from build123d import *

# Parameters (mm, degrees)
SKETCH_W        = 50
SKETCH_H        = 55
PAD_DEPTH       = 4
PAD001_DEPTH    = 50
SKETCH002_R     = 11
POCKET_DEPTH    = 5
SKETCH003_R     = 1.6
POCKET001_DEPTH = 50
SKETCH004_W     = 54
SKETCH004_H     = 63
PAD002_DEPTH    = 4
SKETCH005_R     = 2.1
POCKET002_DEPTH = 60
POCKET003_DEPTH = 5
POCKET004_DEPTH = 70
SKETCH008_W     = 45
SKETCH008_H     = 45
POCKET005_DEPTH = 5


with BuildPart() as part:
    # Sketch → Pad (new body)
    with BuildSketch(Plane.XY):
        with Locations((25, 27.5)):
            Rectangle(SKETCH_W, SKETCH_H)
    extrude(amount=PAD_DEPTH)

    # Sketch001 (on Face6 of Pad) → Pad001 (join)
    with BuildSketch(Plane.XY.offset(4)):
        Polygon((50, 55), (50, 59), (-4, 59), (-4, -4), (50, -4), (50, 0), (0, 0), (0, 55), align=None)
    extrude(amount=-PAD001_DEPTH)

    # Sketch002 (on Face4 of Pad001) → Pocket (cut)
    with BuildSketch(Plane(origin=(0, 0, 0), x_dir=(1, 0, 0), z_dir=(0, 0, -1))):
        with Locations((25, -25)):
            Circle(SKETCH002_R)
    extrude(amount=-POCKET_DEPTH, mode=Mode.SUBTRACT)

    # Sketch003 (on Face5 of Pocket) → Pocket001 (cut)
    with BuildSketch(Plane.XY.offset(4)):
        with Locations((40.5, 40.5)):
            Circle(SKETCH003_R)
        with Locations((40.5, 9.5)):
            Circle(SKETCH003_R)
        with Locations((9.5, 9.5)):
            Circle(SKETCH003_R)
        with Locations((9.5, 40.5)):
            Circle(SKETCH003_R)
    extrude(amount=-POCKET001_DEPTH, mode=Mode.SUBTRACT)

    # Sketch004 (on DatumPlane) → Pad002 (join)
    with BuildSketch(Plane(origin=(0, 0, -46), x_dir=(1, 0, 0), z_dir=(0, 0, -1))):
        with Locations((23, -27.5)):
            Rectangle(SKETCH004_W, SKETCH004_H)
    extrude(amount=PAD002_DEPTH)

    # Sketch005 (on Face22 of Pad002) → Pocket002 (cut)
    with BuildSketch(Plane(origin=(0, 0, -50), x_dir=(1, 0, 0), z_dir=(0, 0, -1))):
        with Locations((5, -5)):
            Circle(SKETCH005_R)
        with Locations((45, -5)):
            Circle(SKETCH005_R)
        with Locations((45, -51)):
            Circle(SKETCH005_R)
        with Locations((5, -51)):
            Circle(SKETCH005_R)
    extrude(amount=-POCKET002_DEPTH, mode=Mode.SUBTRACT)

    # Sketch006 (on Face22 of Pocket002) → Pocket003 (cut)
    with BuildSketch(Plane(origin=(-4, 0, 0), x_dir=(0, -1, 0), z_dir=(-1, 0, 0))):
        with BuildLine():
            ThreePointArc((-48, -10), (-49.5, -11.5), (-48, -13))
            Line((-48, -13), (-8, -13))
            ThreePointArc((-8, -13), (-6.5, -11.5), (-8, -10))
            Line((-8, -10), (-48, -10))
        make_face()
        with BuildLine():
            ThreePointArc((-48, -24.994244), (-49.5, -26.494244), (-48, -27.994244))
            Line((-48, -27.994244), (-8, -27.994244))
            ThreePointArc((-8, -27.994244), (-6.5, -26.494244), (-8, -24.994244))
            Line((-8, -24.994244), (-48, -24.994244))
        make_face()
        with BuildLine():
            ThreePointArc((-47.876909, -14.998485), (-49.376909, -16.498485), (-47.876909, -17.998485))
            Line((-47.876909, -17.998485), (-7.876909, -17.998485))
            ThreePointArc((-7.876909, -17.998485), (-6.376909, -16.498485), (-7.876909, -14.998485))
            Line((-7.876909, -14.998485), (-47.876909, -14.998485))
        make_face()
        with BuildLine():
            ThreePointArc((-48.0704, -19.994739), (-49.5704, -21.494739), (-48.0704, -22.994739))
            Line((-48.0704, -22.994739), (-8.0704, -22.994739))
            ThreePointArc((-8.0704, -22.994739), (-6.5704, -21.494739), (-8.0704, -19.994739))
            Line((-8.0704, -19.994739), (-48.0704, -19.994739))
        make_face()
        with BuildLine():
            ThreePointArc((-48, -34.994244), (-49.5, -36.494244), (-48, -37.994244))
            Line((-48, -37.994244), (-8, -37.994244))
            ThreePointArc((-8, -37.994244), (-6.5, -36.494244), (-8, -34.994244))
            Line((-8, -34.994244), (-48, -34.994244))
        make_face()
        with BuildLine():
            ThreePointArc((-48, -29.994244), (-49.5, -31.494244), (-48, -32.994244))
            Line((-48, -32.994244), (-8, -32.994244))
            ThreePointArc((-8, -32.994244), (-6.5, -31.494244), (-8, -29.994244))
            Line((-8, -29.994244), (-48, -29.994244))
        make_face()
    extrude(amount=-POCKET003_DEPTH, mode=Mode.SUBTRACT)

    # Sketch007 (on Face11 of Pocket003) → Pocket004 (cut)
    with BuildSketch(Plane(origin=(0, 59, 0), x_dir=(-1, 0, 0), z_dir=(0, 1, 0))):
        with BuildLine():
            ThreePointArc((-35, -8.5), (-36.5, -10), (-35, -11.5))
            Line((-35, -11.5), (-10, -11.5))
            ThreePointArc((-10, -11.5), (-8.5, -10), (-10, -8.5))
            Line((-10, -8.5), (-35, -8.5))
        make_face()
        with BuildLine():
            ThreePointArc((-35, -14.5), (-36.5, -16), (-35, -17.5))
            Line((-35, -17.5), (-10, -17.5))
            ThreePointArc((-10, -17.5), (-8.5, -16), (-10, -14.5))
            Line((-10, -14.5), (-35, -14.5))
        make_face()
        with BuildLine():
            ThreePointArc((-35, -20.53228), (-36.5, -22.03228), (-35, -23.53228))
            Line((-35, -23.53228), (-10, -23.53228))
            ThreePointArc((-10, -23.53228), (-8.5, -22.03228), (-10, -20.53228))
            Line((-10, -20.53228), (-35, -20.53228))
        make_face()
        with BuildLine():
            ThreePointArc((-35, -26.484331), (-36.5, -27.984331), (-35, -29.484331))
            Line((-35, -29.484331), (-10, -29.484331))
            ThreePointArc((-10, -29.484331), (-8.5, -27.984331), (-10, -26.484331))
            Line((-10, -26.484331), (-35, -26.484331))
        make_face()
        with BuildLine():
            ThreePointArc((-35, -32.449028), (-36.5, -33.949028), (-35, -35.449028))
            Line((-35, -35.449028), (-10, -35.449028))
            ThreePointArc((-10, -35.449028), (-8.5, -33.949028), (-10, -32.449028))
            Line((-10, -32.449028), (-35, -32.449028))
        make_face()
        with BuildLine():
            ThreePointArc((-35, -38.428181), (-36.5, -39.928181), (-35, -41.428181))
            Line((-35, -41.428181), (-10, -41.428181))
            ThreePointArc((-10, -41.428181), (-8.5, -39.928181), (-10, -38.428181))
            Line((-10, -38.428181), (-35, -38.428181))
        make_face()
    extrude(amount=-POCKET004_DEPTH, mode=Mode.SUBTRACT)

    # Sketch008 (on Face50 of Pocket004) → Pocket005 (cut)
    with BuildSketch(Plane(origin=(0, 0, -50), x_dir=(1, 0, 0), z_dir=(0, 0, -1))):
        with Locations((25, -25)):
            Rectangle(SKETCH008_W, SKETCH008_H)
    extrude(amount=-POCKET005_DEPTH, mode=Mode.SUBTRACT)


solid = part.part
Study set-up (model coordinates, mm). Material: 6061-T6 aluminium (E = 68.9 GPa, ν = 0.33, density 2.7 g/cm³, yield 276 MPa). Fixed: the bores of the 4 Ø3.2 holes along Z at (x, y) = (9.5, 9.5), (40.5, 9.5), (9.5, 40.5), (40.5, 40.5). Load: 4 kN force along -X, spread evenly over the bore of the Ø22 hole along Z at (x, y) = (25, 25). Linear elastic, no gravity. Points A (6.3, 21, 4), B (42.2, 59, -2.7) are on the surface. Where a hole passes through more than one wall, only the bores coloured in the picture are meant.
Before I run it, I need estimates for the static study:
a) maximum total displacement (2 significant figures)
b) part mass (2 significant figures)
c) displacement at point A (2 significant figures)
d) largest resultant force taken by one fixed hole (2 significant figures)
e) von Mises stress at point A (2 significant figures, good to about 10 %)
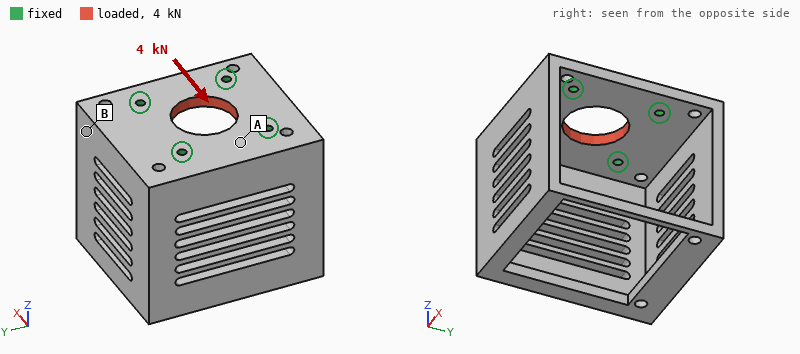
7.0 µm
110 g
4.0 µm
1.0 kN
10 MPa
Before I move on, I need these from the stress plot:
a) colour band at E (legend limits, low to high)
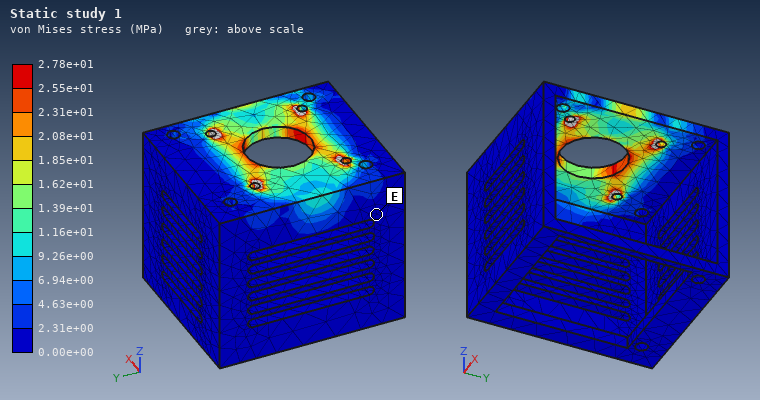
0.00e+00 to 2.31e+00 MPa
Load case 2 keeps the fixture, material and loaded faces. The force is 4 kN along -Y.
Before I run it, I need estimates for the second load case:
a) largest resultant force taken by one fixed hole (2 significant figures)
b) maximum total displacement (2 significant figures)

1.0 kN
5.8 µm
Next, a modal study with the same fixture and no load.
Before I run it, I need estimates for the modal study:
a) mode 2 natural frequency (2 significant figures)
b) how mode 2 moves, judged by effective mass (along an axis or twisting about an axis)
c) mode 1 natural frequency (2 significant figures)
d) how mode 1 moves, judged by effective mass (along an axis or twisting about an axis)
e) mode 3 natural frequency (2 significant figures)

1900 Hz
along X
1300 Hz
along Y
2700 Hz
